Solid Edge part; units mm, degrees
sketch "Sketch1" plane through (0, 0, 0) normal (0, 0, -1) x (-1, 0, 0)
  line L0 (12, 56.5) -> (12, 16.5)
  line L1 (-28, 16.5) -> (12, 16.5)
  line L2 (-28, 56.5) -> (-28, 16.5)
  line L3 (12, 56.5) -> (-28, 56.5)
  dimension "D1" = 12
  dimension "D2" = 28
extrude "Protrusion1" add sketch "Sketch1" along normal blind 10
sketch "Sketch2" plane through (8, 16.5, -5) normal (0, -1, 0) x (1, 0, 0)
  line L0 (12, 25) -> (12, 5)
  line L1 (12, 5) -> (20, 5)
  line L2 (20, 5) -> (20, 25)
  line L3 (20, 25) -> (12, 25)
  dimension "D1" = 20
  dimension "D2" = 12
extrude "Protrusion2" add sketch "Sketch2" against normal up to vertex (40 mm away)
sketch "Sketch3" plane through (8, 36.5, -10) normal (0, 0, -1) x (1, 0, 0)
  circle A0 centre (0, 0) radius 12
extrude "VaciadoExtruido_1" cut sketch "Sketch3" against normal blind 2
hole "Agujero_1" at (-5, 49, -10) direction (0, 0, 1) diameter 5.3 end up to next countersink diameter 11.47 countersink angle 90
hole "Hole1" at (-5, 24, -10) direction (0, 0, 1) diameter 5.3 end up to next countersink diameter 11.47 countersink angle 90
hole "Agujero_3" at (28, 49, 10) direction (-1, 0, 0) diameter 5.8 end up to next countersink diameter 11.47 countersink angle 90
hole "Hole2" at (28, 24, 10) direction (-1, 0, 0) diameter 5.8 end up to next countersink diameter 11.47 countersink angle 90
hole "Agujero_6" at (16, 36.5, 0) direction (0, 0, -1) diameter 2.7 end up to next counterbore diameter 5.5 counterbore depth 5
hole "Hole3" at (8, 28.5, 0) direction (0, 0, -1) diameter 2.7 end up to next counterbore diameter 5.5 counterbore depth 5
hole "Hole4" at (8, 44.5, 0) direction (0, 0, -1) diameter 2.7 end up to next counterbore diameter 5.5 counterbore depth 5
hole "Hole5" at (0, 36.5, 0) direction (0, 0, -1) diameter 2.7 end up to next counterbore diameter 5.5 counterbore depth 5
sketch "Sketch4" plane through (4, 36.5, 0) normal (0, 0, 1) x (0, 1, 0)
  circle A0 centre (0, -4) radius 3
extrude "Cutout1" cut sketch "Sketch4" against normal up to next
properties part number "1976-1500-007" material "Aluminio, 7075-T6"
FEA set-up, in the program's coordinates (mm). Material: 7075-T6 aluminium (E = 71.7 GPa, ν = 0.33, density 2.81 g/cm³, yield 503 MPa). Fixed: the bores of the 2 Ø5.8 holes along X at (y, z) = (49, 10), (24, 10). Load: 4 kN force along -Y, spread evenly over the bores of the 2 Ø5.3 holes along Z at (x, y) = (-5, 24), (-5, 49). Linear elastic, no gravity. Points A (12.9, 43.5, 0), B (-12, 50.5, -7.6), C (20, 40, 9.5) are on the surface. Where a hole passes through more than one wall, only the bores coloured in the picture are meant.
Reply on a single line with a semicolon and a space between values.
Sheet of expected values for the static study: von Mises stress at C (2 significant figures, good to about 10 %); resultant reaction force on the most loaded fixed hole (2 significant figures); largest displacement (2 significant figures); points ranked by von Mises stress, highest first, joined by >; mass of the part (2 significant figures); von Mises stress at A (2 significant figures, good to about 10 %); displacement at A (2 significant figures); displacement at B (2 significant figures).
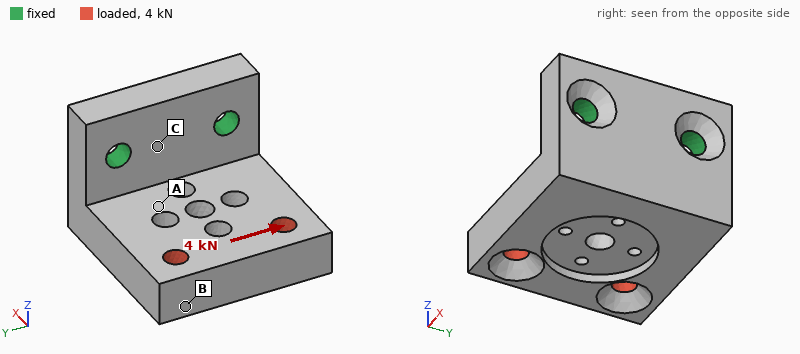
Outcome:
54 MPa; 4.6 kN; 0.20 mm; A > C > B; 55 g; 88 MPa; 0.061 mm; 0.17 mm
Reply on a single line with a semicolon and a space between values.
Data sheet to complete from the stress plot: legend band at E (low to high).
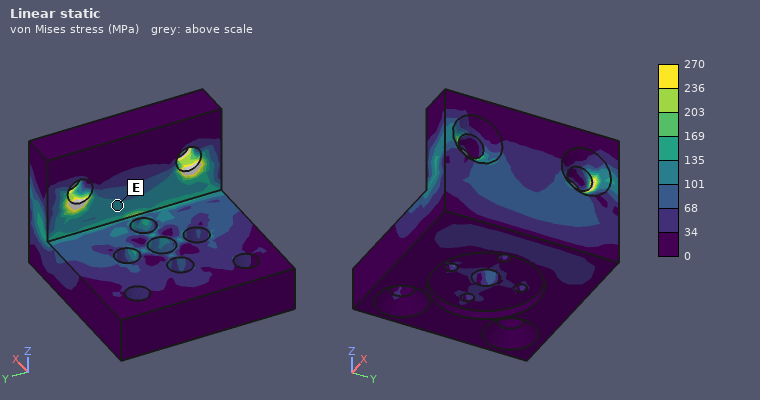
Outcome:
101 to 135 MPa
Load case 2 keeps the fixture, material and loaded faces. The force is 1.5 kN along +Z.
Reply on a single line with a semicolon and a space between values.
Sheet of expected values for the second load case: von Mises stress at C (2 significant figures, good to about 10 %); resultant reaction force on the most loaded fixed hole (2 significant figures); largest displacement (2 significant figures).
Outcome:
53 MPa; 790 N; 0.31 mm
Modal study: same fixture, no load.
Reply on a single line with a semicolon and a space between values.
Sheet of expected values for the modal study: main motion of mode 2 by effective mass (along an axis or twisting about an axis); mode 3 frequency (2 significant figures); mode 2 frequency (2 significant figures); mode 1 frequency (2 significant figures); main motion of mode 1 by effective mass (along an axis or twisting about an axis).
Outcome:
along Y; 9500 Hz; 5700 Hz; 2900 Hz; along Z
